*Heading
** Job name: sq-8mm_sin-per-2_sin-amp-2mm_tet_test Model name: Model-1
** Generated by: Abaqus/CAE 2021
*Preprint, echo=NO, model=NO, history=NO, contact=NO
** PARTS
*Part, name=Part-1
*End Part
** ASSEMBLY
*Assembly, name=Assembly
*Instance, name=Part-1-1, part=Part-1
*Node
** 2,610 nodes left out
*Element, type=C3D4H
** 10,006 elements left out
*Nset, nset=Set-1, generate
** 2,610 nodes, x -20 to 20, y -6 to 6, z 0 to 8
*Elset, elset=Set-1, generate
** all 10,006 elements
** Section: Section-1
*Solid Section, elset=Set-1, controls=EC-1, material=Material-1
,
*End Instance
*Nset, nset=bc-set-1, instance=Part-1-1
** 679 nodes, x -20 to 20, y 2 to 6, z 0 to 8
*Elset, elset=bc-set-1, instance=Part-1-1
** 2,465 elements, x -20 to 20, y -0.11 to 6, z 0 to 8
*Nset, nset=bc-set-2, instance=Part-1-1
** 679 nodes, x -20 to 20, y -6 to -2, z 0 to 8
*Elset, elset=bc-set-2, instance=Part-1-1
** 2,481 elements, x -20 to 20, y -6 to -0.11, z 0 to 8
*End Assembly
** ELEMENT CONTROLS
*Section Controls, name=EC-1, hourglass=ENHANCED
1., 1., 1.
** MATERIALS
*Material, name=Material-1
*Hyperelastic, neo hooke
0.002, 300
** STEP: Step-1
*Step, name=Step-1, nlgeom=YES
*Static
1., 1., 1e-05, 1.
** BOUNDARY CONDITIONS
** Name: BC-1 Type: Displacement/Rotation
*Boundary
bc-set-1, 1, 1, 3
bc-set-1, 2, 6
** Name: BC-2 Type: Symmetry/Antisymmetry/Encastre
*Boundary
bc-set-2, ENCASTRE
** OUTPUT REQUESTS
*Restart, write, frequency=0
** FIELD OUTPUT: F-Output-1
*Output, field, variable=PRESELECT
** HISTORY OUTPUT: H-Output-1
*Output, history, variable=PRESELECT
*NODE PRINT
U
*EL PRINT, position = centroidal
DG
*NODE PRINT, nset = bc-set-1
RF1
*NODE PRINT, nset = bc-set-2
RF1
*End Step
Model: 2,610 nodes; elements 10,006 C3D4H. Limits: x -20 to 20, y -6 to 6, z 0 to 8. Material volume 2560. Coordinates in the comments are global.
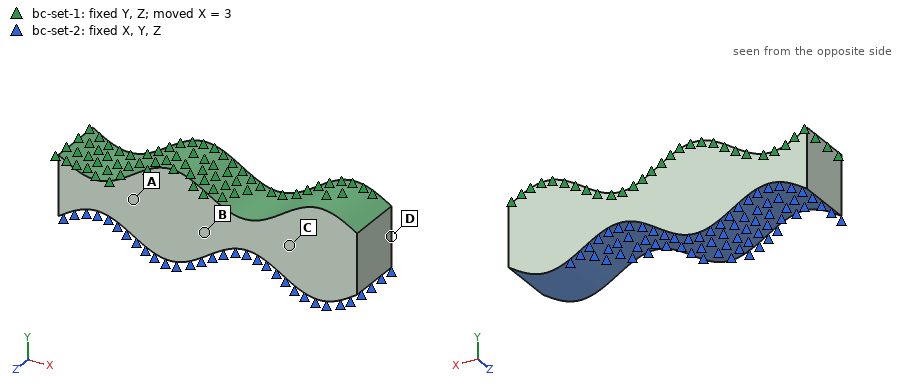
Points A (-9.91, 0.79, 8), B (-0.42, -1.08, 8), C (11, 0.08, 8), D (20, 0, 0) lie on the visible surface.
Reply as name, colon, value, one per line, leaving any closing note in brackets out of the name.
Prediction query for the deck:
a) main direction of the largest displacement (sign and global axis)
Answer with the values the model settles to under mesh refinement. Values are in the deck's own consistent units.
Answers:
main direction of the largest displacement: +X
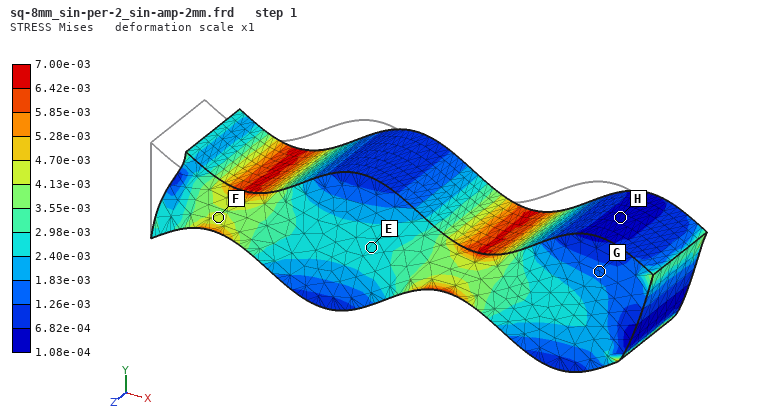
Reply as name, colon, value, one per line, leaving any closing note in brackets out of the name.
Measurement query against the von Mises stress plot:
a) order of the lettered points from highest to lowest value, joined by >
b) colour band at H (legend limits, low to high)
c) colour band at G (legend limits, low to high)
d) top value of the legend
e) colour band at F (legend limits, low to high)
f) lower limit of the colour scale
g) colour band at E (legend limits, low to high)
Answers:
order of the lettered points from highest to lowest value, joined by >: F > E > G > H
colour band at H: 1.08e-04 to 6.82e-04
colour band at G: 1.26e-03 to 1.83e-03
top value of the legend: 7.00e-03
colour band at F: 4.13e-03 to 4.70e-03
lower limit of the colour scale: 1.08e-04
colour band at E: 2.40e-03 to 2.98e-03
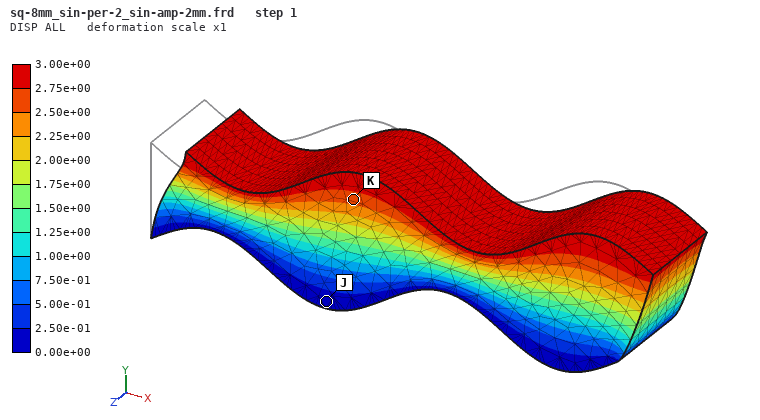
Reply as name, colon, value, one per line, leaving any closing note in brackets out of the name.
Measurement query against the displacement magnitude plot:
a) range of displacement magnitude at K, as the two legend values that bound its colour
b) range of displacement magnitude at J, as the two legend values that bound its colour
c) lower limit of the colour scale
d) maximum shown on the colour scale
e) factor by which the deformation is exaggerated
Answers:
range of displacement magnitude at K, as the two legend values that bound its colour: 2.50e+00 to 2.75e+00
range of displacement magnitude at J, as the two legend values that bound its colour: 0.00e+00 to 2.50e-01
lower limit of the colour scale: 0.00e+00
maximum shown on the colour scale: 3.00e+00
factor by which the deformation is exaggerated: 1
